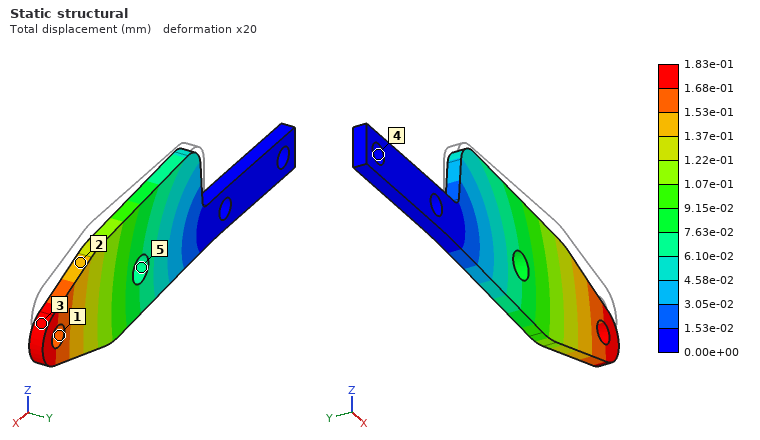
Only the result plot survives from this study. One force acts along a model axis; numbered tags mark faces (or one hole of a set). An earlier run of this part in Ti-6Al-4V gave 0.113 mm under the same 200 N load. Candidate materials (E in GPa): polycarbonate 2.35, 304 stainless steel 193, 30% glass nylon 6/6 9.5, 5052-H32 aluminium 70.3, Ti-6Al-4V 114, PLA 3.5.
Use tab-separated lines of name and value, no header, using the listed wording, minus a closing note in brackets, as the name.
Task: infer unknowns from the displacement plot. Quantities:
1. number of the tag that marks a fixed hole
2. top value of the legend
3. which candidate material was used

number of the tag that marks a fixed hole	4
top value of the legend	1.83e-01 mm
which candidate material was used	5052-H32 aluminium
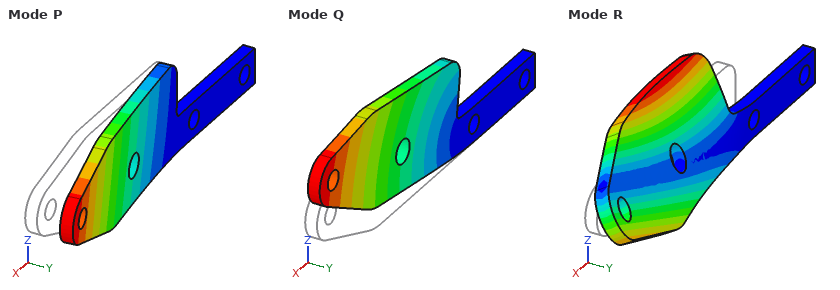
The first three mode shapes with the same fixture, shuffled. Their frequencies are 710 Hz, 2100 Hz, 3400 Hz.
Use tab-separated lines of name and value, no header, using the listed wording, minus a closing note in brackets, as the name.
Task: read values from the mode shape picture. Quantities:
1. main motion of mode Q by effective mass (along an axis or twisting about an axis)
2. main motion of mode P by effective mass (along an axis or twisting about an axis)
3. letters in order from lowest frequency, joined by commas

main motion of mode Q by effective mass	along Z
main motion of mode P by effective mass	along Y
letters in order from lowest frequency, joined by commas	P, Q, R
